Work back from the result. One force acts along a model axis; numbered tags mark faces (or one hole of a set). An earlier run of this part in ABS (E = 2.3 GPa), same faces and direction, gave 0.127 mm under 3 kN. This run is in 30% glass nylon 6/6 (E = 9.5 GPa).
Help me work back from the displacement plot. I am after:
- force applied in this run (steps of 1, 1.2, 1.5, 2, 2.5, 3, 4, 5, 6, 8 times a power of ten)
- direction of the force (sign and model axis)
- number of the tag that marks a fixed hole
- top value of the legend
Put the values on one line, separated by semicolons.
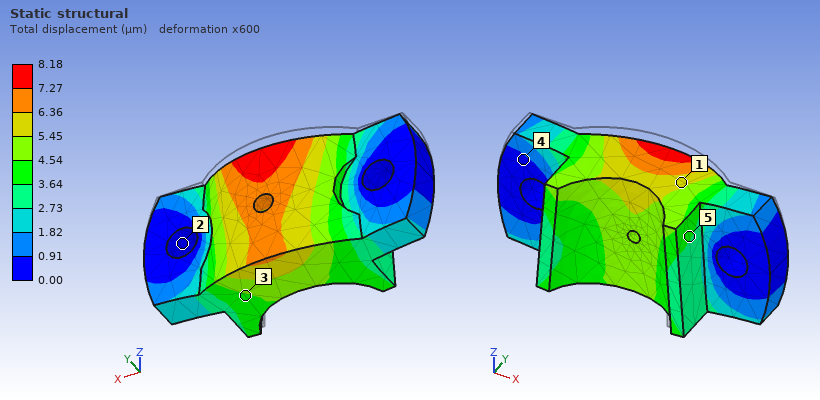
800 N; -Z; 2; 8.18 µm
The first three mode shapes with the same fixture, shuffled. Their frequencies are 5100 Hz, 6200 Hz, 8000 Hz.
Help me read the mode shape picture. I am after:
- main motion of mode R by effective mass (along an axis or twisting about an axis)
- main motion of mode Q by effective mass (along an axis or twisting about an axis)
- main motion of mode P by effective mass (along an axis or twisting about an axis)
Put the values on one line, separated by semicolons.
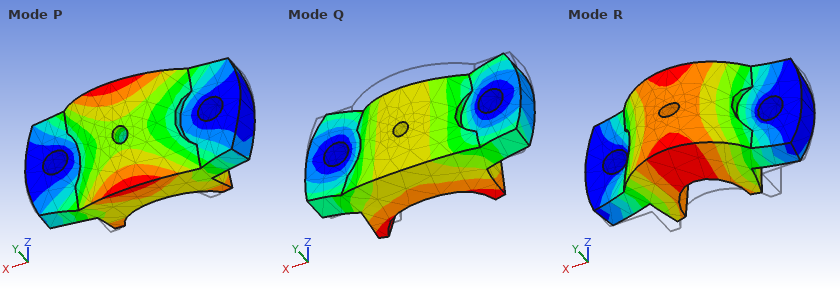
along Y; along Z; twisting about X
